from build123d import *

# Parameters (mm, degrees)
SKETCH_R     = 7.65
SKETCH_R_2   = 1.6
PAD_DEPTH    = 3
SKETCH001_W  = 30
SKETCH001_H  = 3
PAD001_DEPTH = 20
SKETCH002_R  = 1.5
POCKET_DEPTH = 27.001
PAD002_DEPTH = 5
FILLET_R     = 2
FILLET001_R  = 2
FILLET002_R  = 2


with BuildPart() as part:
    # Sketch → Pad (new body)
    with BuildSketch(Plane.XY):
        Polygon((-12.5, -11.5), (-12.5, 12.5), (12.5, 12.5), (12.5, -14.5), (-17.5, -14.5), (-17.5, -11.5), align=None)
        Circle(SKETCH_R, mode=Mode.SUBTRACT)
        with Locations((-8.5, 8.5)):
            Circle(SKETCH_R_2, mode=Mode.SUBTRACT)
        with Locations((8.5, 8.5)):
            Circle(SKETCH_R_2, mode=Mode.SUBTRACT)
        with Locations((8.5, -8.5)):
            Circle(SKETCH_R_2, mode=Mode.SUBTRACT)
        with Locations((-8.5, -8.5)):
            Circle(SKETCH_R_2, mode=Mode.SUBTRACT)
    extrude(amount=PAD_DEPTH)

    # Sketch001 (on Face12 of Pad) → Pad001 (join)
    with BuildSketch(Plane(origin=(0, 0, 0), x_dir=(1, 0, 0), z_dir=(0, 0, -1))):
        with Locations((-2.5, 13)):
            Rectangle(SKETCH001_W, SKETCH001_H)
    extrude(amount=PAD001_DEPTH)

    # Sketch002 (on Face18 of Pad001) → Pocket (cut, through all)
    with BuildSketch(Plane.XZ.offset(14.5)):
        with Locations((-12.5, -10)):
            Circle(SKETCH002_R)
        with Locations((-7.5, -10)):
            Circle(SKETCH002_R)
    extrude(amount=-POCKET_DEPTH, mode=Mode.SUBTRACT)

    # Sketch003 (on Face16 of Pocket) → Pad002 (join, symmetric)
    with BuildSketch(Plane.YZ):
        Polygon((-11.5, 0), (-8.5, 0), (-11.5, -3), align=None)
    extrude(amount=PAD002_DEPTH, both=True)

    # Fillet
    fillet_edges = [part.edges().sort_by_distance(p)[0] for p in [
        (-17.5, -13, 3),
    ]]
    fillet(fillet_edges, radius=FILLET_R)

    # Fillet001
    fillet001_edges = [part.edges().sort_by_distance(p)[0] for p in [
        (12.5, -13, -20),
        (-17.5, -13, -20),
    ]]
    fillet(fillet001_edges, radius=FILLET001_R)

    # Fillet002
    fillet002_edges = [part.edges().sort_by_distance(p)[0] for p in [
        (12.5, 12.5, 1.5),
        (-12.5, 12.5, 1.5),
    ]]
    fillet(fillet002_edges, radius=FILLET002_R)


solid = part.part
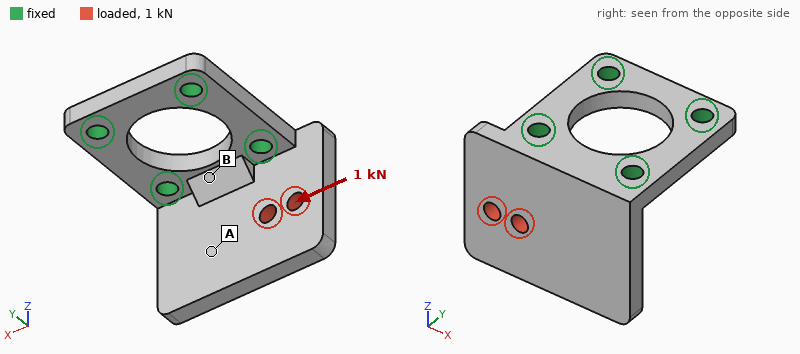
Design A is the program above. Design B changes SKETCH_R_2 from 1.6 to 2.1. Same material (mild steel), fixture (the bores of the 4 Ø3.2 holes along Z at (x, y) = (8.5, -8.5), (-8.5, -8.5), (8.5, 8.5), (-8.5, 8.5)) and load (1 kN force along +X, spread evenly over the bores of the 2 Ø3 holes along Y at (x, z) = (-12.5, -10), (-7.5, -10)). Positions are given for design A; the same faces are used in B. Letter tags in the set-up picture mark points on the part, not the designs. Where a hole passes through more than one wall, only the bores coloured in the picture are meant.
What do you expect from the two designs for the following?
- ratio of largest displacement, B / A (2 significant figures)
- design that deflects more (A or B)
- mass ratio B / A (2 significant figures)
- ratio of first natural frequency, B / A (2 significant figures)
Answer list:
0.81
A
0.98
1.1
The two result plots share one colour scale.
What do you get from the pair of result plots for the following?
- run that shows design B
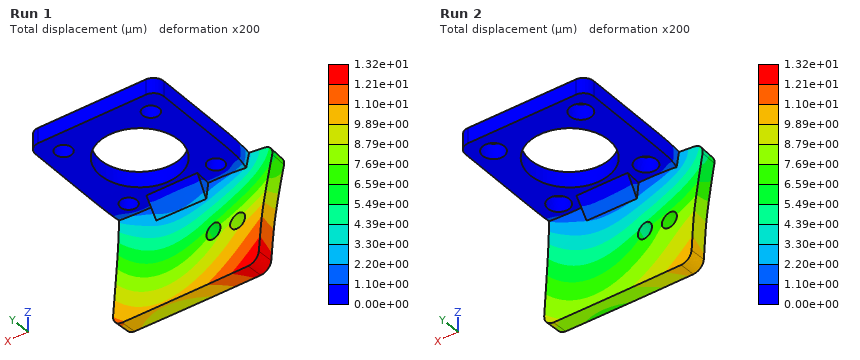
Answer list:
Run 2
